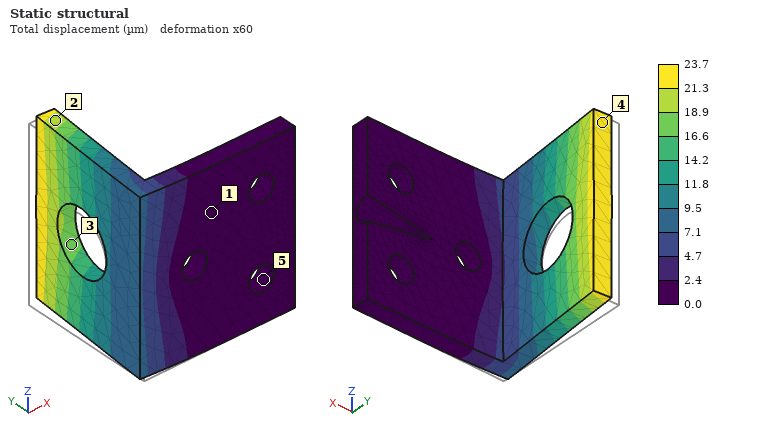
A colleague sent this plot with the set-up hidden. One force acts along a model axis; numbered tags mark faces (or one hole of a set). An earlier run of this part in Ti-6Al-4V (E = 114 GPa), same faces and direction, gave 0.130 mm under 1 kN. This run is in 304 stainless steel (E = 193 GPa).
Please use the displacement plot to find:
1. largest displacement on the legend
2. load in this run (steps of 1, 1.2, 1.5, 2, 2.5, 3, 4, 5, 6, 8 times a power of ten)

23.7 µm
300 N
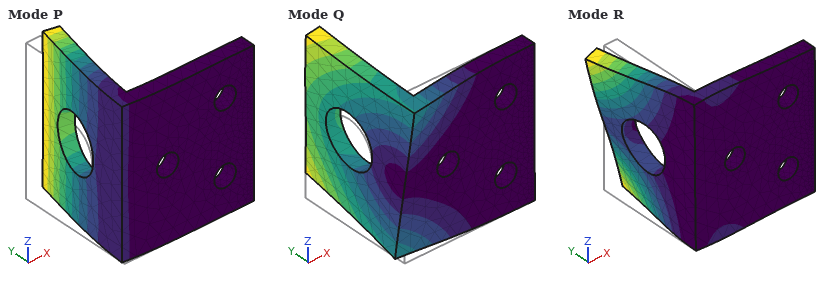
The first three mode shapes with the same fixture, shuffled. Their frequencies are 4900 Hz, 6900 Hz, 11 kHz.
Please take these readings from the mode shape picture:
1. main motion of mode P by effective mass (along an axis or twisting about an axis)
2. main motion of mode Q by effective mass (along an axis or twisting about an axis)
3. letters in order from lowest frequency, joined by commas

along X
along Z
P, Q, R
